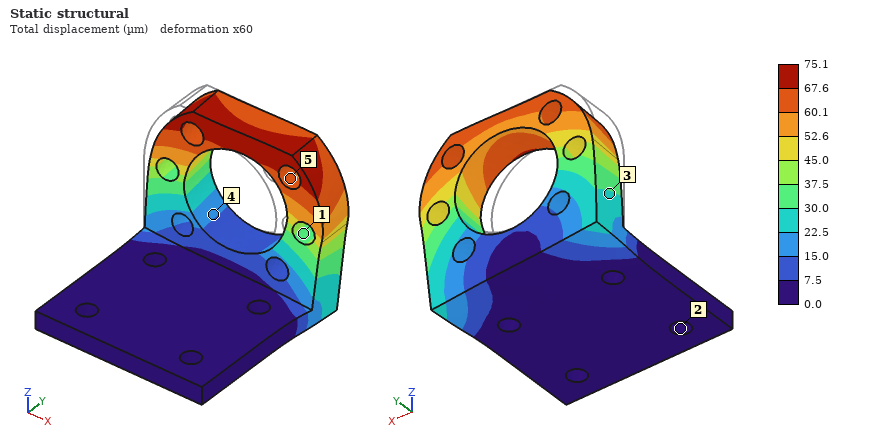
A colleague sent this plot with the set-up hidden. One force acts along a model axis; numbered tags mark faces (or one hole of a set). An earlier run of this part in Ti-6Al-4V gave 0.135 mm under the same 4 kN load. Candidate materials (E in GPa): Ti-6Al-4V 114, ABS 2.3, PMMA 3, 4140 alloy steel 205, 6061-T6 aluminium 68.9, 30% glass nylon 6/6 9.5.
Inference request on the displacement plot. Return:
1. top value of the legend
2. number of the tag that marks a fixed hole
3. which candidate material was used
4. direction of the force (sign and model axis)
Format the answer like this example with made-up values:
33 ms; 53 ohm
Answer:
75.1 µm; 2; 4140 alloy steel; +X
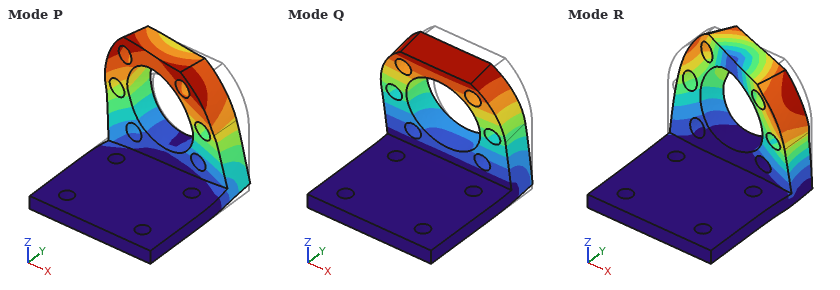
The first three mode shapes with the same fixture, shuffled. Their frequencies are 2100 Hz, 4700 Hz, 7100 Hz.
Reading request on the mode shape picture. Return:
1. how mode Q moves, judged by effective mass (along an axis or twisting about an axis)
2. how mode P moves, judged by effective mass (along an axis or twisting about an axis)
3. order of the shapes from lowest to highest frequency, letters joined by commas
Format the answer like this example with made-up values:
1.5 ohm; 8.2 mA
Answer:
along Y; along X; Q, P, R
